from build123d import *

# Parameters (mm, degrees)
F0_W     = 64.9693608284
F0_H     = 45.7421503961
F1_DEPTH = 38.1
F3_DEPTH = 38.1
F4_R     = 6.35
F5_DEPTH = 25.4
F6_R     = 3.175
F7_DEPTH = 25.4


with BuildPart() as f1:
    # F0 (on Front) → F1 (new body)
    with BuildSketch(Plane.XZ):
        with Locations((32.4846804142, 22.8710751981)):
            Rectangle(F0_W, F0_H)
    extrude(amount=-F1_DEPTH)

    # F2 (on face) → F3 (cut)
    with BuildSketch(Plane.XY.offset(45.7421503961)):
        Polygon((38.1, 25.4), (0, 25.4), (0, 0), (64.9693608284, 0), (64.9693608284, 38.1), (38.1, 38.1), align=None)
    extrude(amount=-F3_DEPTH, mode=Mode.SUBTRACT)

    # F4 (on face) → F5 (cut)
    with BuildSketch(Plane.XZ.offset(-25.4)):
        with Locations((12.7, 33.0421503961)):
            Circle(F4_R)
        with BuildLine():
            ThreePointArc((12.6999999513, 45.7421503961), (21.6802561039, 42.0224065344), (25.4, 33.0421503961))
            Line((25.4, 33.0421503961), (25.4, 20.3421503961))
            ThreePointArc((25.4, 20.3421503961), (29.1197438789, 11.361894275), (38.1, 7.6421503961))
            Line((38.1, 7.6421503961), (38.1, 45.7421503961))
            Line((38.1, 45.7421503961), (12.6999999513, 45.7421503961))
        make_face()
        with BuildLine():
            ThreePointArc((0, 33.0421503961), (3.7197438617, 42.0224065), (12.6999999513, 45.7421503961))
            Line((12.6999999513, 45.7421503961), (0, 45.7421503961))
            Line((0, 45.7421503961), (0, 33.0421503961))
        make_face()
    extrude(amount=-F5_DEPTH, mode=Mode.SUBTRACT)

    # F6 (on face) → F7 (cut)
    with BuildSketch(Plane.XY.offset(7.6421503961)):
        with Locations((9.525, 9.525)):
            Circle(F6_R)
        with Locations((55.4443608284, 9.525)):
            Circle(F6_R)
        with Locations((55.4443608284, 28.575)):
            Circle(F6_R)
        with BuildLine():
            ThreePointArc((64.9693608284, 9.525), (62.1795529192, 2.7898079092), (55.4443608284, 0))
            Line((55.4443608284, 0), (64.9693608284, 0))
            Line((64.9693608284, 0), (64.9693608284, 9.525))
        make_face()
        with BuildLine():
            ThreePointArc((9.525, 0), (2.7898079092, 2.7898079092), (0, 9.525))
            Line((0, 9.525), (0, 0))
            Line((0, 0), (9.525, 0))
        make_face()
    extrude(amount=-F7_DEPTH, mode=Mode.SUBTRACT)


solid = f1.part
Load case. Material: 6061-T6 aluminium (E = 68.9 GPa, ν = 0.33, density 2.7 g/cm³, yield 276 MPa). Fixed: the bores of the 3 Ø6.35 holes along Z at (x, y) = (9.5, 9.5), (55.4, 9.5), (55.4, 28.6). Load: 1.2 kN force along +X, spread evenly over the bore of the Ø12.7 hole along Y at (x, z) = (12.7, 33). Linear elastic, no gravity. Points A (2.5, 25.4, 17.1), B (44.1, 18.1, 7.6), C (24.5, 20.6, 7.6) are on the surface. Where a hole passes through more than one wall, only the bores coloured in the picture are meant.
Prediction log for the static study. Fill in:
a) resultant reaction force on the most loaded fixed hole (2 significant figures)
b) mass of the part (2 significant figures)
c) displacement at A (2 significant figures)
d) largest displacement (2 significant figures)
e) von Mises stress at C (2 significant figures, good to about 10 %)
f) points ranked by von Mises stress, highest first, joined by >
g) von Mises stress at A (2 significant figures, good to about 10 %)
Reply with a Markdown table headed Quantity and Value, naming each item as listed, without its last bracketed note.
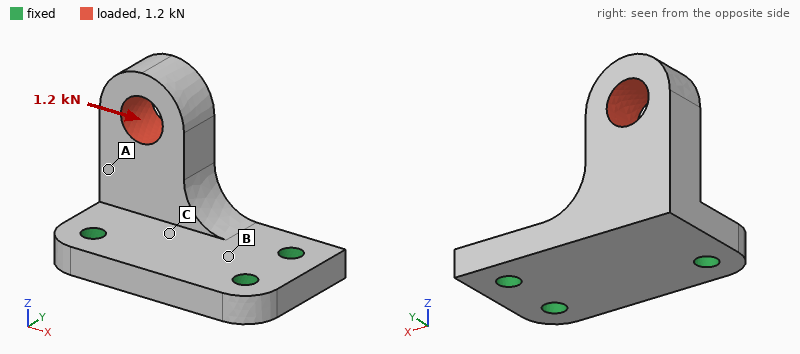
| Quantity | Value |
|---|---|
| resultant reaction force on the most loaded fixed hole | 910 N |
| mass of the part | 76 g |
| displacement at A | 43 µm |
| largest displacement | 96 µm |
| von Mises stress at C | 26 MPa |
| points ranked by von Mises stress, highest first, joined by > | C > A > B |
| von Mises stress at A | 14 MPa |
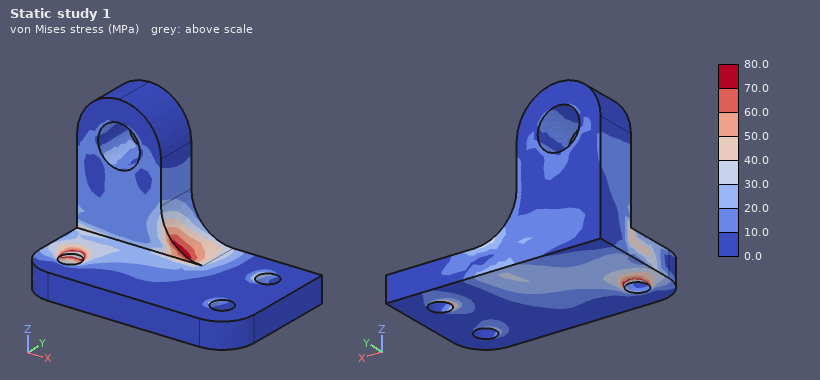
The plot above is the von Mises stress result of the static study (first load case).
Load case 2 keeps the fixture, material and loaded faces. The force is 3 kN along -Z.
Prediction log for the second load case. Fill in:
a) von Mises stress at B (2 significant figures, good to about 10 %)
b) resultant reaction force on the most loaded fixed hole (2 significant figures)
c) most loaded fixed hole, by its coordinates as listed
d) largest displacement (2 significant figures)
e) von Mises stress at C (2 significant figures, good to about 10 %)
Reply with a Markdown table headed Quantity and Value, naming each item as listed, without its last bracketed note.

| Quantity | Value |
|---|---|
| von Mises stress at B | 37 MPa |
| resultant reaction force on the most loaded fixed hole | 2.5 kN |
| most loaded fixed hole, by its coordinates as listed | (9.5, 9.5) |
| largest displacement | 0.25 mm |
| von Mises stress at C | 51 MPa |
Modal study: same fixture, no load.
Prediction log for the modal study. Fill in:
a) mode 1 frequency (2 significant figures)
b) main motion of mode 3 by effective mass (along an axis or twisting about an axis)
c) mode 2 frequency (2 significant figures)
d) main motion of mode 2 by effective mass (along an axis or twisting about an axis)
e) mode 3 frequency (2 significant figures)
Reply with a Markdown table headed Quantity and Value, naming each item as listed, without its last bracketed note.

| Quantity | Value |
|---|---|
| mode 1 frequency | 2800 Hz |
| main motion of mode 3 by effective mass | along Z |
| mode 2 frequency | 5600 Hz |
| main motion of mode 2 by effective mass | along X |
| mode 3 frequency | 8500 Hz |
